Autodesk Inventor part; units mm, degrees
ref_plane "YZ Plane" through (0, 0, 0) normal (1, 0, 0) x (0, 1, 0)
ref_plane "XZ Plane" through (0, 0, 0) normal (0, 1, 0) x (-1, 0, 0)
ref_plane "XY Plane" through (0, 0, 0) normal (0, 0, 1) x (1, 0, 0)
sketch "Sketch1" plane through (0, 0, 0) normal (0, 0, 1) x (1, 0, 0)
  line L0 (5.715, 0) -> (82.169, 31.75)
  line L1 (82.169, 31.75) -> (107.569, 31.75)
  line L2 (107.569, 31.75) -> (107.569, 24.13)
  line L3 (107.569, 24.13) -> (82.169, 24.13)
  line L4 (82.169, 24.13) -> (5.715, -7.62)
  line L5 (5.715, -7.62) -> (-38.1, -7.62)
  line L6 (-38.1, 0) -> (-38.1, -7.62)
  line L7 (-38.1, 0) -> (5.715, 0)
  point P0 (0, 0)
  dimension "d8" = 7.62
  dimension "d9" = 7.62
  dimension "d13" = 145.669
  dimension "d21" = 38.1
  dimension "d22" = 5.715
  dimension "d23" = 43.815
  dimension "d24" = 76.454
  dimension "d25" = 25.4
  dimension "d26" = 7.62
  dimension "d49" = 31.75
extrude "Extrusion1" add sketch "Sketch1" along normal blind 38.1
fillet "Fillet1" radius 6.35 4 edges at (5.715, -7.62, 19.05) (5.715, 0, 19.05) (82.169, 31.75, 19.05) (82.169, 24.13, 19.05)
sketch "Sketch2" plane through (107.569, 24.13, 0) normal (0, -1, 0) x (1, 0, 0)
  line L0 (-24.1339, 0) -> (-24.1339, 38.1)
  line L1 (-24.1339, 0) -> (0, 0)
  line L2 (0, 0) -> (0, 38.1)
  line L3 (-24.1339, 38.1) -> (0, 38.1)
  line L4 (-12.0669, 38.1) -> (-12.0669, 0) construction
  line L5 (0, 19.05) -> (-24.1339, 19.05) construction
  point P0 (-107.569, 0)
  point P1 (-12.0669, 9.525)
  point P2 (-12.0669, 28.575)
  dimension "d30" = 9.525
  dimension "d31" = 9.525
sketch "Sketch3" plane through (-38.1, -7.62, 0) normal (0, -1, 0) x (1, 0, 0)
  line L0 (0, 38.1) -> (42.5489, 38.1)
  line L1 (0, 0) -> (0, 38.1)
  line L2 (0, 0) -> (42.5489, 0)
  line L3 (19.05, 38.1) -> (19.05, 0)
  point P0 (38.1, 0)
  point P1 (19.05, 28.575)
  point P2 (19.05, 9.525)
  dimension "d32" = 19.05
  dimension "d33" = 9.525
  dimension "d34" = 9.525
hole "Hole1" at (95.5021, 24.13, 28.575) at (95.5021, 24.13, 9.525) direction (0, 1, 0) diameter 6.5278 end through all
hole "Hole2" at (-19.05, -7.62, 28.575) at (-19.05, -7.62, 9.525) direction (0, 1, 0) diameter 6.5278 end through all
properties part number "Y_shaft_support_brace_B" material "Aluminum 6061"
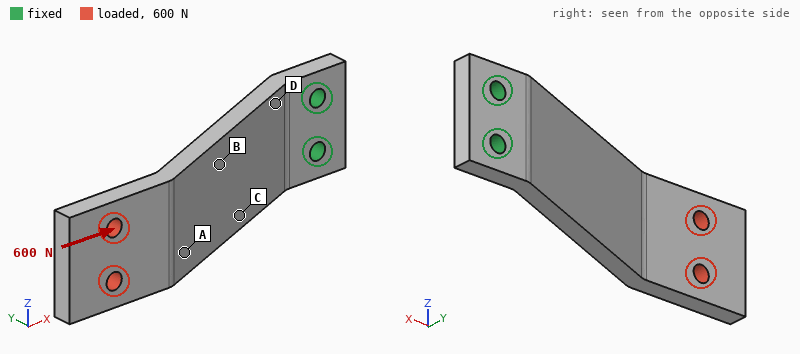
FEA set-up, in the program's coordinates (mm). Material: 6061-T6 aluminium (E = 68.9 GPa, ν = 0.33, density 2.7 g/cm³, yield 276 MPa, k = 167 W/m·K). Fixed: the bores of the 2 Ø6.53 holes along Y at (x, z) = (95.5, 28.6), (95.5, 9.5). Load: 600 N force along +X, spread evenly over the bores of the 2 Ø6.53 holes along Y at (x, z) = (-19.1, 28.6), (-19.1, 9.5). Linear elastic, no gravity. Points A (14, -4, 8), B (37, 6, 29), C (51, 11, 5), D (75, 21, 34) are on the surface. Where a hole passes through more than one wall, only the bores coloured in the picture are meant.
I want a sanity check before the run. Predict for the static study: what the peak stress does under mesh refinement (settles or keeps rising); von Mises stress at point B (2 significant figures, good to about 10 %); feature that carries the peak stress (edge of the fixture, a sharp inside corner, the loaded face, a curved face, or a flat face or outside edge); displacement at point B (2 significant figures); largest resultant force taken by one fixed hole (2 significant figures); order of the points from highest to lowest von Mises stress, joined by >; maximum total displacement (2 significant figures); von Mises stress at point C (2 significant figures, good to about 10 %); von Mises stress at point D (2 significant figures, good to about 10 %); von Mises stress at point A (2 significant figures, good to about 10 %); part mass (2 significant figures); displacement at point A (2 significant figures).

keeps rising
26 MPa
edge of the fixture
0.37 mm
320 N
D > C > B > A
1.3 mm
37 MPa
54 MPa
8.3 MPa
110 g
0.67 mm
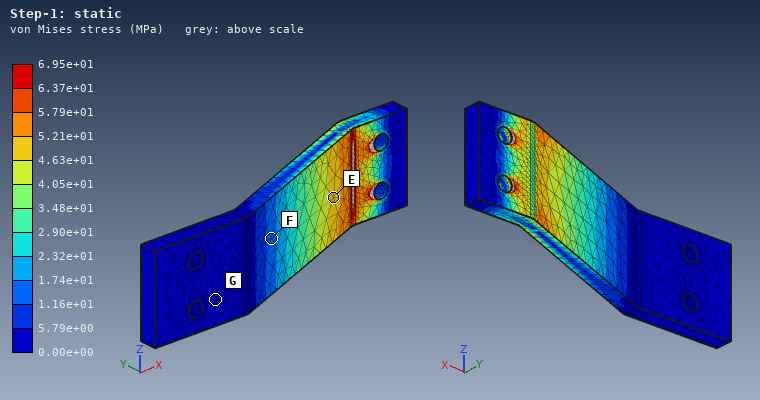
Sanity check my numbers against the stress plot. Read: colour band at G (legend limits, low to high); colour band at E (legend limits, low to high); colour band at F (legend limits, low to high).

0.00e+00 to 5.79e+00 MPa
4.63e+01 to 5.21e+01 MPa
1.16e+01 to 1.74e+01 MPa
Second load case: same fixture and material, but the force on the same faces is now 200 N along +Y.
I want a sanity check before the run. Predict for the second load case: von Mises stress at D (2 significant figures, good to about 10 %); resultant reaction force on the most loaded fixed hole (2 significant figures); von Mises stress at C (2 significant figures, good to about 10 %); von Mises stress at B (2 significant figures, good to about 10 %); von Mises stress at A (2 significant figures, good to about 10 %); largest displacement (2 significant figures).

57 MPa
130 N
43 MPa
35 MPa
20 MPa
1.6 mm
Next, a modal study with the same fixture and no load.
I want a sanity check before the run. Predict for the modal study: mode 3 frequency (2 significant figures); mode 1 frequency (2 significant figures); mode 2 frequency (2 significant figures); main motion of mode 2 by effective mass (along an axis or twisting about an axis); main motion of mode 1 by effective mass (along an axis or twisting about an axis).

1900 Hz
310 Hz
1300 Hz
along Z
along Y
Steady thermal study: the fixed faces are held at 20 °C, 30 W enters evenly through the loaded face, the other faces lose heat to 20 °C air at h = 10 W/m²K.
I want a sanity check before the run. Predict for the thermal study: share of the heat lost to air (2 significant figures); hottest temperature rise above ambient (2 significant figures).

17 %
71 K
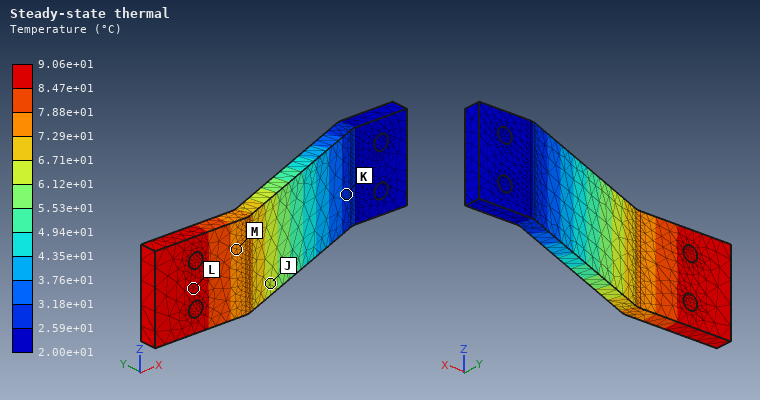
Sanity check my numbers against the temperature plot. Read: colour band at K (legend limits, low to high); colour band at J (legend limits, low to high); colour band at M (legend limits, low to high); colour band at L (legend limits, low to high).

2.59e+01 to 3.18e+01 °C
6.12e+01 to 6.71e+01 °C
7.29e+01 to 7.88e+01 °C
8.47e+01 to 9.06e+01 °C
